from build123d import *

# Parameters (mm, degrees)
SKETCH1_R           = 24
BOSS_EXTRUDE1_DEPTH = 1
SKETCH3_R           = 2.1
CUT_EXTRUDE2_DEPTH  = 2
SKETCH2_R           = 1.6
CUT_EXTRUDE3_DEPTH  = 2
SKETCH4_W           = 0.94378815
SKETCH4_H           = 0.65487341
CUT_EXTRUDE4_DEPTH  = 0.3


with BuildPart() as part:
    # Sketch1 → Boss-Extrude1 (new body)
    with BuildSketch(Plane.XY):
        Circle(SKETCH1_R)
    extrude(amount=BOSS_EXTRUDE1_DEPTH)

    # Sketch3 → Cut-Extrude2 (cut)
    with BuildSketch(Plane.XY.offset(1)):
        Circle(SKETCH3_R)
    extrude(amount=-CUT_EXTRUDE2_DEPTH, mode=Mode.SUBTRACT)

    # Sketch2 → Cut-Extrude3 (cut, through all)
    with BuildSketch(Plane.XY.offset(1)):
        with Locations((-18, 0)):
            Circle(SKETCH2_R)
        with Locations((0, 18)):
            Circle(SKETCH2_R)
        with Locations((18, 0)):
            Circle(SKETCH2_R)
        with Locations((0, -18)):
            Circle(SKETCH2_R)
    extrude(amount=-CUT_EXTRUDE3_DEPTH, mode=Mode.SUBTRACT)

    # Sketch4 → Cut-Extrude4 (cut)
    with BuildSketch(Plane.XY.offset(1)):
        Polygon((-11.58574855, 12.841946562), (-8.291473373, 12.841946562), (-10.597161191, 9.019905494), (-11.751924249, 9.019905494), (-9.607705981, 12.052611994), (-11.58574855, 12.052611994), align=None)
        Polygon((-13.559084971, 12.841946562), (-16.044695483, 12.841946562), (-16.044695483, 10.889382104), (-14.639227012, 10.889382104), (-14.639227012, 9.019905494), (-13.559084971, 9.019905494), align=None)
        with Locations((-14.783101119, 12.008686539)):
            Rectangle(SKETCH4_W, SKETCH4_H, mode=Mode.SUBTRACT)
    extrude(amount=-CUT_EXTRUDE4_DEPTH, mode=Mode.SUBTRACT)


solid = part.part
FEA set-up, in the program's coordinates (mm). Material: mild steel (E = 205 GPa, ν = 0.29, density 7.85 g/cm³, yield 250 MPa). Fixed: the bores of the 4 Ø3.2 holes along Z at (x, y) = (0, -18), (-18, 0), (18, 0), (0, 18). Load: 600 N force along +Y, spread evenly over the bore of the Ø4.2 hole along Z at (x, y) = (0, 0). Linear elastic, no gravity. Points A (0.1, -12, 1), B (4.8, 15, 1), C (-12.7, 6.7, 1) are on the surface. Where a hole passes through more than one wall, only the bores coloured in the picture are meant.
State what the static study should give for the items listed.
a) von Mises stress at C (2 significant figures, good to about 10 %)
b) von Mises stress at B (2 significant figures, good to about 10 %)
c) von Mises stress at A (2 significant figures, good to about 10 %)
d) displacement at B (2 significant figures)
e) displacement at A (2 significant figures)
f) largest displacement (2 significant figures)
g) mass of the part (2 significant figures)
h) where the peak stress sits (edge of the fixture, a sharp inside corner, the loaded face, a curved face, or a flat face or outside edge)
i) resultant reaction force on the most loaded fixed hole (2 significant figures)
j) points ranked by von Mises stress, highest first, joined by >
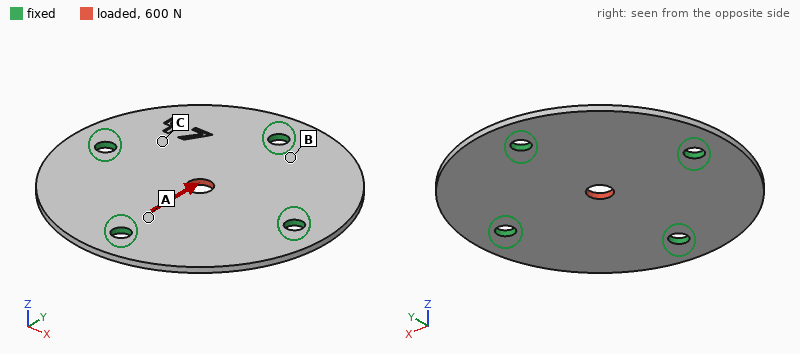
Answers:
5.5 MPa
10 MPa
25 MPa
0.51 µm
0.59 µm
2.0 µm
14 g
the loaded face
200 N
A > B > C
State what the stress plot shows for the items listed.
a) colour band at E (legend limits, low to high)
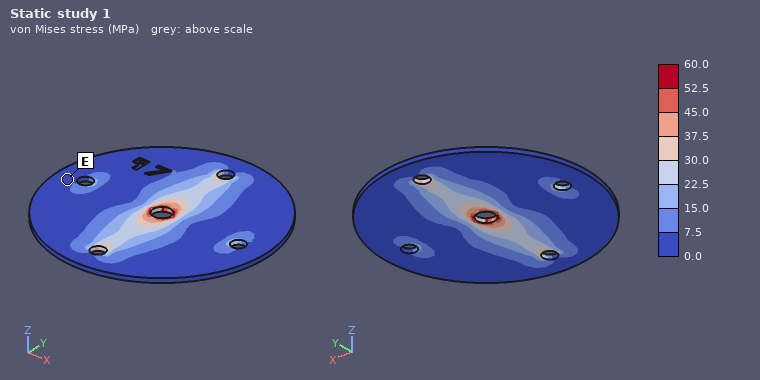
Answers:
0.0 to 7.5 MPa
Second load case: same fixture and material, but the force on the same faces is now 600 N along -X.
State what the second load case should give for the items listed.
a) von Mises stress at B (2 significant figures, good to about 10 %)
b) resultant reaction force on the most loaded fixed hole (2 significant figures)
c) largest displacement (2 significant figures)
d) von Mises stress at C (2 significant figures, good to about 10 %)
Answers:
6.7 MPa
200 N
2.0 µm
8.4 MPa
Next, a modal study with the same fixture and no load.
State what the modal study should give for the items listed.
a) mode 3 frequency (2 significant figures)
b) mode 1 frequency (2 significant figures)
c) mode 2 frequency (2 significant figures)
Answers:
6200 Hz
6000 Hz
6200 Hz
